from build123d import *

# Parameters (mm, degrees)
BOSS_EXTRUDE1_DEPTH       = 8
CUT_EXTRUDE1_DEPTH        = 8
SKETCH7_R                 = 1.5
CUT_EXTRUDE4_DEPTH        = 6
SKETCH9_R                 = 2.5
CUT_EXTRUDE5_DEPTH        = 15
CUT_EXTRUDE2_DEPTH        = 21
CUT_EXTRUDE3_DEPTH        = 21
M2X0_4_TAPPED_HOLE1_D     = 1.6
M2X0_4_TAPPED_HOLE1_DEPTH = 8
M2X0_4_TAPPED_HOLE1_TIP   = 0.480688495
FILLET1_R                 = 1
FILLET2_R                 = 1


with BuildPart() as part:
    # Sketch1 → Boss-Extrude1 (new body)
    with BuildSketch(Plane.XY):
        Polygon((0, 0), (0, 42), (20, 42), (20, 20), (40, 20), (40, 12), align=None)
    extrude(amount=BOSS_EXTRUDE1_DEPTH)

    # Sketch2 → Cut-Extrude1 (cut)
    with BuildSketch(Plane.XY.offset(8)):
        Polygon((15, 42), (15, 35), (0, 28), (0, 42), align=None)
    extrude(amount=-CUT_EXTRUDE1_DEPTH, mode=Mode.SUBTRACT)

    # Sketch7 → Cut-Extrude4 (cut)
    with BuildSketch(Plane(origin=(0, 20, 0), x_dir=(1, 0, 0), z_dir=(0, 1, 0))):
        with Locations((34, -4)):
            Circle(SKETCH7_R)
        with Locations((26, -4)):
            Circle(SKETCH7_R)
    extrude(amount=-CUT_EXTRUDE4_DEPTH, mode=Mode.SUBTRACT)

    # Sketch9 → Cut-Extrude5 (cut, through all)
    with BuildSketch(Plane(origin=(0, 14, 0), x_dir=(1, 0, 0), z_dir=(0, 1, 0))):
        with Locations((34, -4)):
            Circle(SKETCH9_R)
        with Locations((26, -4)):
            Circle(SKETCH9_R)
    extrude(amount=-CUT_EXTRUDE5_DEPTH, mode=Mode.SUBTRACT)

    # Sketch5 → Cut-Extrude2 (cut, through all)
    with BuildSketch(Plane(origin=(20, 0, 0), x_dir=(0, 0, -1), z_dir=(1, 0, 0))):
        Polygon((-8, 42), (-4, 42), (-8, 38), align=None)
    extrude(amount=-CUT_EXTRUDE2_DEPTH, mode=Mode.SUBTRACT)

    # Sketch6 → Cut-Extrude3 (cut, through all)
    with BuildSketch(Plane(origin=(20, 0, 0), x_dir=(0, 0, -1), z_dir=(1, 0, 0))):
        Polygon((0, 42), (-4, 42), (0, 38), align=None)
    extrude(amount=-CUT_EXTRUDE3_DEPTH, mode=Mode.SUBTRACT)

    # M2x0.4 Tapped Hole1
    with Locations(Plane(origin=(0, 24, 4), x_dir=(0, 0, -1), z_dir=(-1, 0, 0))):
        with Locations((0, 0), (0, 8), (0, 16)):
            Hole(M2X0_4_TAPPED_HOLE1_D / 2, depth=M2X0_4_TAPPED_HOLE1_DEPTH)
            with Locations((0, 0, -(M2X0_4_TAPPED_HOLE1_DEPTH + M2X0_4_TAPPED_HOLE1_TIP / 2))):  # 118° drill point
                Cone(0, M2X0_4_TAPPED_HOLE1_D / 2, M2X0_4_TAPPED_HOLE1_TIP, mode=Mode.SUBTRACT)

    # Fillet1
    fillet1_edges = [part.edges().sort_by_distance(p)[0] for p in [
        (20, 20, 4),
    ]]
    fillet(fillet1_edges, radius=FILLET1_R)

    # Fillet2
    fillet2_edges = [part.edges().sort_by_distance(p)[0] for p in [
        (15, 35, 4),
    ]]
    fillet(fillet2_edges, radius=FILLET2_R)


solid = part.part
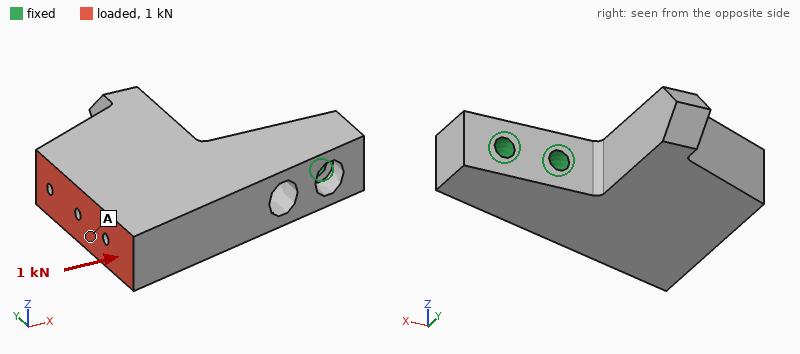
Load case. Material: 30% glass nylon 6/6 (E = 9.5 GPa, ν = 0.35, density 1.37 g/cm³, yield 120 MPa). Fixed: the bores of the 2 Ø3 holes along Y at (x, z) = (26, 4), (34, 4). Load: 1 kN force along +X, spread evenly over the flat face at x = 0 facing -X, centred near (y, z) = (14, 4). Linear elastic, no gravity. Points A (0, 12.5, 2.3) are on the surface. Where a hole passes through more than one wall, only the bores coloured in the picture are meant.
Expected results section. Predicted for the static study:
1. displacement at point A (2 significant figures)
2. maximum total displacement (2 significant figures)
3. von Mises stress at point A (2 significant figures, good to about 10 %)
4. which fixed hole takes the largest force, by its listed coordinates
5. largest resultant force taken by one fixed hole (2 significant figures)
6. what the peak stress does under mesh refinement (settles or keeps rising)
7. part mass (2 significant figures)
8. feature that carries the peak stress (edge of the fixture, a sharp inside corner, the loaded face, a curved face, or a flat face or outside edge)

67 µm
95 µm
6.4 MPa
(26, 4)
780 N
keeps rising
8.7 g
edge of the fixture
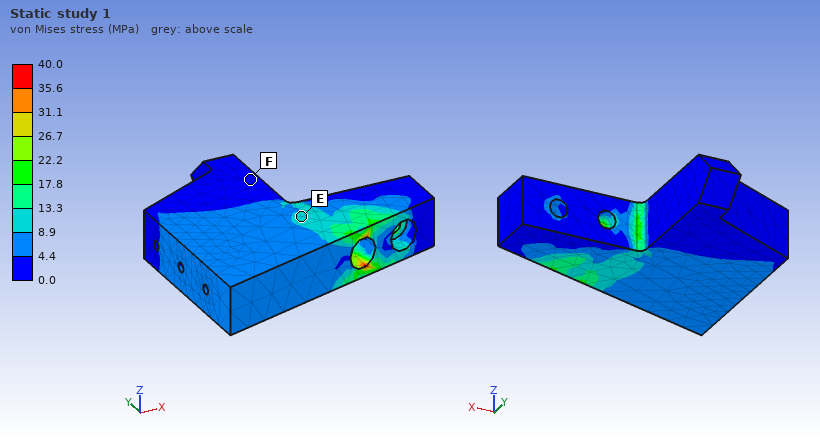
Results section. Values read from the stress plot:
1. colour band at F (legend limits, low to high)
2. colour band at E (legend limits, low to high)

0.0 to 4.4 MPa
8.9 to 13.3 MPa
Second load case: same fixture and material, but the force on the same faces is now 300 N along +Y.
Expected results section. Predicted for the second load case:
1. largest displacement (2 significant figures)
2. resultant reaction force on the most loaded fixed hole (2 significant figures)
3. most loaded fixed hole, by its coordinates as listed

0.31 mm
760 N
(26, 4)
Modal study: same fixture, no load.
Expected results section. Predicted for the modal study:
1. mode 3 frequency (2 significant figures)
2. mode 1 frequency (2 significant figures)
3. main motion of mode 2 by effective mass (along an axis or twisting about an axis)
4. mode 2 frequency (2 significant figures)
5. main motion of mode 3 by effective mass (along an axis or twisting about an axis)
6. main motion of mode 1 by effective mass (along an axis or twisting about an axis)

3400 Hz
2500 Hz
along Y
2900 Hz
twisting about X
along Z
